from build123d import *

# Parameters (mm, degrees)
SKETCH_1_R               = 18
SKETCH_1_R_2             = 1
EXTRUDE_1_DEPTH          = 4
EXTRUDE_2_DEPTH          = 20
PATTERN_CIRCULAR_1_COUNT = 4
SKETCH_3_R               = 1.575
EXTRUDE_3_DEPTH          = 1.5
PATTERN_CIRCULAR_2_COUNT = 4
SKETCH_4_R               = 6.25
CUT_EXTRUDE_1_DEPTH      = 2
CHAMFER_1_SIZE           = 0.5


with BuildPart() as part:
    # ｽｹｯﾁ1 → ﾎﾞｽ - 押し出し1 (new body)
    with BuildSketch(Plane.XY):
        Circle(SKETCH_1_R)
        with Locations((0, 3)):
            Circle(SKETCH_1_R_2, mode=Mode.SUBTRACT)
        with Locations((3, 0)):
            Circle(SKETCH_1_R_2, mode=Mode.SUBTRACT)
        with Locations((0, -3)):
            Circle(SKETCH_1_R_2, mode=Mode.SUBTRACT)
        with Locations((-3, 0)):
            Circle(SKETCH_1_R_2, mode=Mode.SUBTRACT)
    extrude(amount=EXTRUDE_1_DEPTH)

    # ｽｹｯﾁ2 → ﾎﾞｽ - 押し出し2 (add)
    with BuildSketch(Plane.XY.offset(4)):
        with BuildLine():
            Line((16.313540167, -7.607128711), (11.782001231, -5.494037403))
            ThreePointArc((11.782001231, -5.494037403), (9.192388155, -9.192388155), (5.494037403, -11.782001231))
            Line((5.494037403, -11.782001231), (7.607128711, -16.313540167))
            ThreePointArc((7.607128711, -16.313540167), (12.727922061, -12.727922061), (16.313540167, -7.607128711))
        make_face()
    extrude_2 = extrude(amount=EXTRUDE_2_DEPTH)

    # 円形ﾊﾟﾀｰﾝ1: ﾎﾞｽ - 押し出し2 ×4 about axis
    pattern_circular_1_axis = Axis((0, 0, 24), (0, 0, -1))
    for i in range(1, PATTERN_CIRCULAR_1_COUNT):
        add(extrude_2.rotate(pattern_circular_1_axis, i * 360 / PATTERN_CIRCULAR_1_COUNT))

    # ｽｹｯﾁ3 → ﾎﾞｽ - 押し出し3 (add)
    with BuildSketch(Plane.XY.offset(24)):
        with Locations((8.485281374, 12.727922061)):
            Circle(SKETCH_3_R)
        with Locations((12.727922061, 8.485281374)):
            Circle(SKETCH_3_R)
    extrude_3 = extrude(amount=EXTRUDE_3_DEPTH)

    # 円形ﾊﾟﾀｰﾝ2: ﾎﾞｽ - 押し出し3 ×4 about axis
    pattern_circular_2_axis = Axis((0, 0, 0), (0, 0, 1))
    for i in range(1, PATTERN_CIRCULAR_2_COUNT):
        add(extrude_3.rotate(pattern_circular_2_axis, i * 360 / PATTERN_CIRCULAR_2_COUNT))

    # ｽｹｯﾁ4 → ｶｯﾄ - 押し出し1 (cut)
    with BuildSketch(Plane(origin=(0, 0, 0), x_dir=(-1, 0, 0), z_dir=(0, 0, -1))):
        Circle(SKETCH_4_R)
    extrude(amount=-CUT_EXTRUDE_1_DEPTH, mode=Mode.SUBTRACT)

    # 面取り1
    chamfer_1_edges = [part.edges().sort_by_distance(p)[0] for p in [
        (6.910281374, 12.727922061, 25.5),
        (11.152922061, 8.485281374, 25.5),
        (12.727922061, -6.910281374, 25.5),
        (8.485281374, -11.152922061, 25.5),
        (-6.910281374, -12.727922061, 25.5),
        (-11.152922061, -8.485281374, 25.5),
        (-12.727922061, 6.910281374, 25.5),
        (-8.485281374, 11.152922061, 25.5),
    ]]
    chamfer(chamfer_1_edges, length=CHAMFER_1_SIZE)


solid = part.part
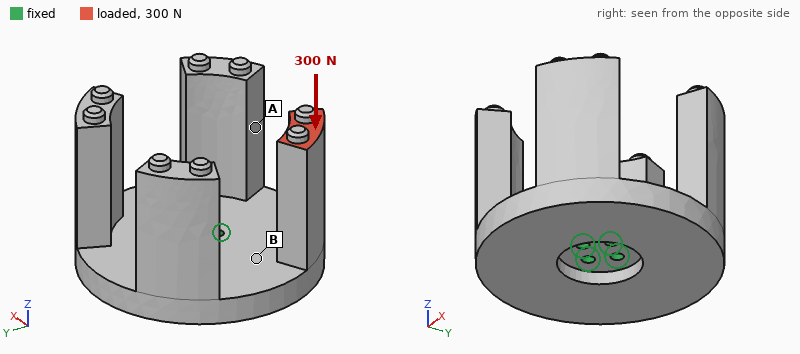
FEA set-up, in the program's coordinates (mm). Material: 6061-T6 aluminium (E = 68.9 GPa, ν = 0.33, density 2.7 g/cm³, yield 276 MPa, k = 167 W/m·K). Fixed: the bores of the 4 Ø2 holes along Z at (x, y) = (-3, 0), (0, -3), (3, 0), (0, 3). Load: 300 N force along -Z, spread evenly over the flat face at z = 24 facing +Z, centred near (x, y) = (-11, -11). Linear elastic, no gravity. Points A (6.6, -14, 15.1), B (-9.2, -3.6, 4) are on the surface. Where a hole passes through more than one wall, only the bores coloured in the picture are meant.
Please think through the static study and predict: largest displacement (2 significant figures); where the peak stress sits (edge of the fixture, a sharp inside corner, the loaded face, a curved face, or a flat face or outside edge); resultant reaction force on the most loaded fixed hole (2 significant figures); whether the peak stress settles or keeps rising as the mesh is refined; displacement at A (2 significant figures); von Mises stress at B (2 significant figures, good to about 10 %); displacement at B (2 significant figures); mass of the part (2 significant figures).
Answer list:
0.15 mm
edge of the fixture
350 N
keeps rising
0.039 mm
28 MPa
0.032 mm
22 g
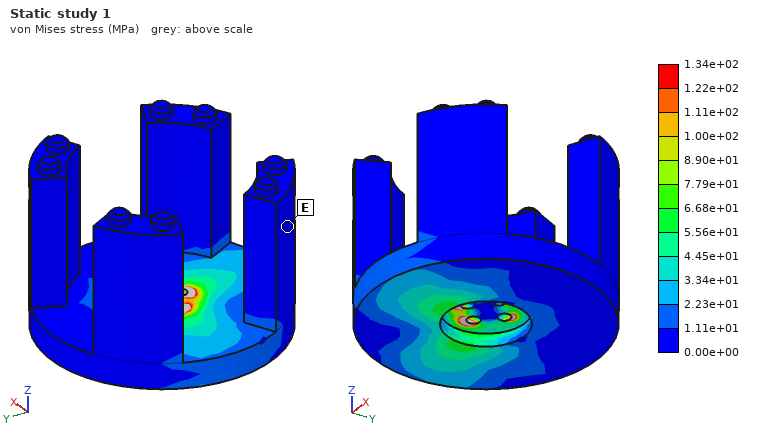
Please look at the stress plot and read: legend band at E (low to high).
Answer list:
0.00e+00 to 1.11e+01 MPa
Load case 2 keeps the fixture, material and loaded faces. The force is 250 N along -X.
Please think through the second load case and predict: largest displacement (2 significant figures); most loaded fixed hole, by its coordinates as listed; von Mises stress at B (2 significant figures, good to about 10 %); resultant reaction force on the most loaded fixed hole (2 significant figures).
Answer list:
0.32 mm
(-3, 0)
51 MPa
560 N
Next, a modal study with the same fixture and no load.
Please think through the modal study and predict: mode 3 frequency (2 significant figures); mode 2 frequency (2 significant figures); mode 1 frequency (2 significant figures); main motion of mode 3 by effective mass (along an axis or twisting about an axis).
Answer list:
4200 Hz
2700 Hz
2700 Hz
along Z
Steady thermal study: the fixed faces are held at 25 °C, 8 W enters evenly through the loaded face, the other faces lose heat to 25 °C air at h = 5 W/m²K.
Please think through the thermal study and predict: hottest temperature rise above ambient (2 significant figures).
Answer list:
28 K
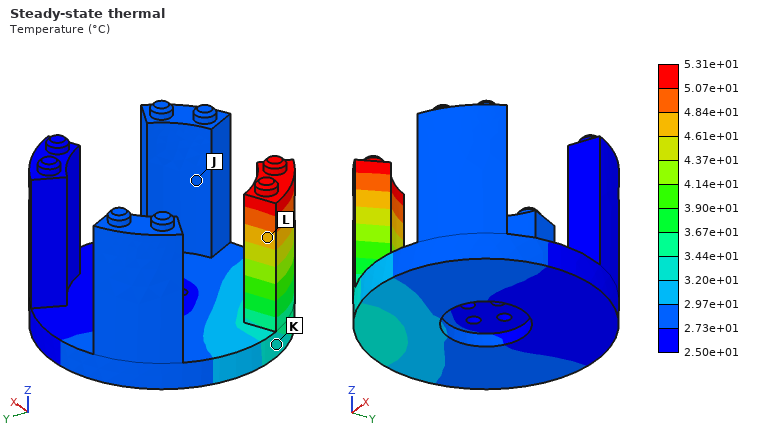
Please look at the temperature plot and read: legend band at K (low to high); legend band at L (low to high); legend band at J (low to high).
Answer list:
3.20e+01 to 3.44e+01 °C
4.61e+01 to 4.84e+01 °C
2.73e+01 to 2.97e+01 °C
